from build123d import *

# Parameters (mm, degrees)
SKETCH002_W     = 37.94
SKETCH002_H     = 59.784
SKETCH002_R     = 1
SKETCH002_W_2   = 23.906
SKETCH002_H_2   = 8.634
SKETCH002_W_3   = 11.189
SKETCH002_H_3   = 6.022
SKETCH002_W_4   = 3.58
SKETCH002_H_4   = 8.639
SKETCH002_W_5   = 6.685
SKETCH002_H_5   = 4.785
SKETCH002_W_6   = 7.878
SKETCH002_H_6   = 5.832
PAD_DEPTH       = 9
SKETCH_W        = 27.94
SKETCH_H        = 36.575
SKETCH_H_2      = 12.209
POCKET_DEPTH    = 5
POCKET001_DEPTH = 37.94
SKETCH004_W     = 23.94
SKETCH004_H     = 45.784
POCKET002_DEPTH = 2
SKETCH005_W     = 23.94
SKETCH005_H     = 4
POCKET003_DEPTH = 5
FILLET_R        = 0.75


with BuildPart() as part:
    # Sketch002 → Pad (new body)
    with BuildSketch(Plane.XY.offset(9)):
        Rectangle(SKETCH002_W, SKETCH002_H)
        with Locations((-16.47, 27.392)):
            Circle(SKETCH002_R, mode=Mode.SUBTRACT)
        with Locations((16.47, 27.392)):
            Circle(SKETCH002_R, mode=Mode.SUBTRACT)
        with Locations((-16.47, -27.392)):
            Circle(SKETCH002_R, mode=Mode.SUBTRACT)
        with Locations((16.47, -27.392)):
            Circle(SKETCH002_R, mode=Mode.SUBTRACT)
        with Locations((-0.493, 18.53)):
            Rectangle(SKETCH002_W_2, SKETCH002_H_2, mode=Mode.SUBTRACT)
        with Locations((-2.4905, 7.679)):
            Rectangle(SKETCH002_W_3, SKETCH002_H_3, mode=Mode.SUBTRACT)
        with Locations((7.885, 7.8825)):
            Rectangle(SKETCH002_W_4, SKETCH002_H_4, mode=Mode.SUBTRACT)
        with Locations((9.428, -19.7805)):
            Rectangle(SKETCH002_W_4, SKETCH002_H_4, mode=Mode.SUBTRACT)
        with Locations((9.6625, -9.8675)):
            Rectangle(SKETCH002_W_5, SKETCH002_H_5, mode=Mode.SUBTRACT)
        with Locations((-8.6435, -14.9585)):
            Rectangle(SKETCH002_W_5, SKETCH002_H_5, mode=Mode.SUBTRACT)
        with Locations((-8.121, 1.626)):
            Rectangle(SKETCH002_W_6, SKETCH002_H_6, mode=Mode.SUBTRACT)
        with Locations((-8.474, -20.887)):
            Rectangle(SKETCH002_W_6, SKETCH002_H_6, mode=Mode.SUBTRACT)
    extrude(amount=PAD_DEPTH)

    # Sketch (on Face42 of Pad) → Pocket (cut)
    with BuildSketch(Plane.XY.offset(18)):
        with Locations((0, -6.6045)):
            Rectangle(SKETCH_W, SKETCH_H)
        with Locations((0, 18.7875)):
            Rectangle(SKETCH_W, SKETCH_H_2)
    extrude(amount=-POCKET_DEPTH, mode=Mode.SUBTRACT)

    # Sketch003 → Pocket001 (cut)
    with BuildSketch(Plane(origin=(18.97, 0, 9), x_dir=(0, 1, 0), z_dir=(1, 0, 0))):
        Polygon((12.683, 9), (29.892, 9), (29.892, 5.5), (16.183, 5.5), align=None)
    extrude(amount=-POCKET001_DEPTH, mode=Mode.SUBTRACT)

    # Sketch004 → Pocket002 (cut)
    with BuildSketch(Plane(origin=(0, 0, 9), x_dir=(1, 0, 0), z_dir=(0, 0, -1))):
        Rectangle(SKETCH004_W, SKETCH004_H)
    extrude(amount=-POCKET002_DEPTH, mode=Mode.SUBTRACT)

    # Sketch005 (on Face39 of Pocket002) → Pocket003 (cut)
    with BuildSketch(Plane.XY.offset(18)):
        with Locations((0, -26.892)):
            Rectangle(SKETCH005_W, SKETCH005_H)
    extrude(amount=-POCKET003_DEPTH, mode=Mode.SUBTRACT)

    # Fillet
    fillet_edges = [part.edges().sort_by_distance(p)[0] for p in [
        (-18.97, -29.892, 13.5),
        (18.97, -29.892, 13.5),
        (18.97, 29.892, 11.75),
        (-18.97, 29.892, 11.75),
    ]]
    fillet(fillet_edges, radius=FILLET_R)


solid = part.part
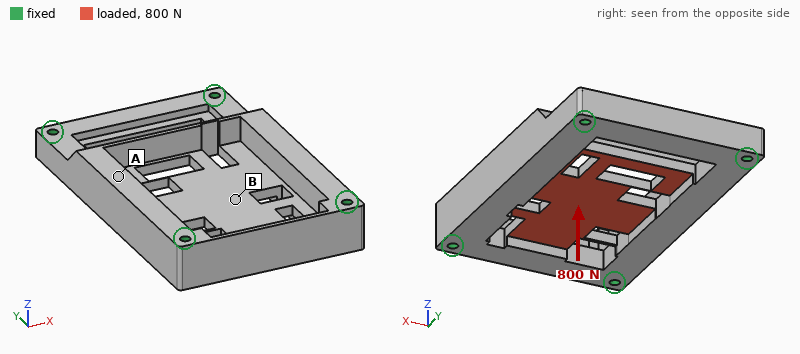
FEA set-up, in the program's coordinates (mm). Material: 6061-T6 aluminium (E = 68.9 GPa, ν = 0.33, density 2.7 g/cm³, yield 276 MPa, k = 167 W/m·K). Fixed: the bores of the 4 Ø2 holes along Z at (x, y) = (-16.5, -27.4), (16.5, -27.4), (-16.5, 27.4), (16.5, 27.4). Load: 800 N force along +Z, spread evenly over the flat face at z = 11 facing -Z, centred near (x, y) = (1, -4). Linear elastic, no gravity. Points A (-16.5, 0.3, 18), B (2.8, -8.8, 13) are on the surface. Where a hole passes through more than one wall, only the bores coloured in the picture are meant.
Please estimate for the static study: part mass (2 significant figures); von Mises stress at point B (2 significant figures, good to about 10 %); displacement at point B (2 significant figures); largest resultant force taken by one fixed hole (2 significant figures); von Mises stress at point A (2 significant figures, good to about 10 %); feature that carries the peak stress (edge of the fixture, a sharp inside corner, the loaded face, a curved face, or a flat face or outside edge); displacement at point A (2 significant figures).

24 g
43 MPa
63 µm
280 N
20 MPa
a flat face or outside edge
20 µm
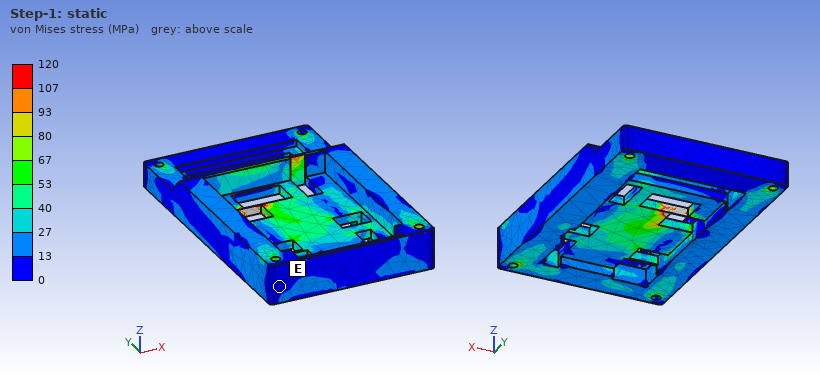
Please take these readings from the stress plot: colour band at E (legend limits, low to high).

0 to 13 MPa
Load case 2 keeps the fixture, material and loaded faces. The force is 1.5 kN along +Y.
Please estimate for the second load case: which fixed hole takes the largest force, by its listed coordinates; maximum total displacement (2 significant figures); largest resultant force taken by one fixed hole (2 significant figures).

(16.5, -27.4)
15 µm
560 N
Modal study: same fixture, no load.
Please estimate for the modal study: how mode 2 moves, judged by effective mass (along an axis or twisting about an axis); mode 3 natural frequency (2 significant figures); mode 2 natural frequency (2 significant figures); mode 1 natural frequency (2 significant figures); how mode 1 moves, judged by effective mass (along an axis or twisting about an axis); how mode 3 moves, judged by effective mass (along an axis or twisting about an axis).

along X
12 kHz
11 kHz
8700 Hz
along Z
along X
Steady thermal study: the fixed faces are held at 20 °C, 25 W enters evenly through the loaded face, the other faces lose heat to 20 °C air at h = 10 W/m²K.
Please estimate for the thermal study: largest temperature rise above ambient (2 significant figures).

24 K
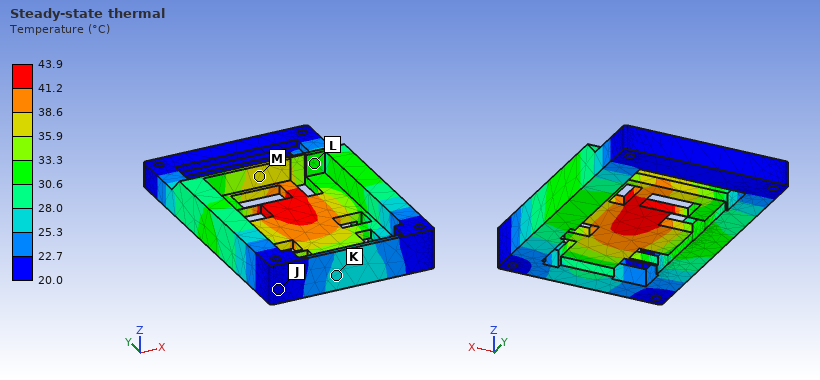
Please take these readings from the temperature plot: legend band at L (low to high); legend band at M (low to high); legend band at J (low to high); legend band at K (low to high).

30.6 to 33.3 °C
35.9 to 38.6 °C
20.0 to 22.7 °C
25.3 to 28.0 °C
